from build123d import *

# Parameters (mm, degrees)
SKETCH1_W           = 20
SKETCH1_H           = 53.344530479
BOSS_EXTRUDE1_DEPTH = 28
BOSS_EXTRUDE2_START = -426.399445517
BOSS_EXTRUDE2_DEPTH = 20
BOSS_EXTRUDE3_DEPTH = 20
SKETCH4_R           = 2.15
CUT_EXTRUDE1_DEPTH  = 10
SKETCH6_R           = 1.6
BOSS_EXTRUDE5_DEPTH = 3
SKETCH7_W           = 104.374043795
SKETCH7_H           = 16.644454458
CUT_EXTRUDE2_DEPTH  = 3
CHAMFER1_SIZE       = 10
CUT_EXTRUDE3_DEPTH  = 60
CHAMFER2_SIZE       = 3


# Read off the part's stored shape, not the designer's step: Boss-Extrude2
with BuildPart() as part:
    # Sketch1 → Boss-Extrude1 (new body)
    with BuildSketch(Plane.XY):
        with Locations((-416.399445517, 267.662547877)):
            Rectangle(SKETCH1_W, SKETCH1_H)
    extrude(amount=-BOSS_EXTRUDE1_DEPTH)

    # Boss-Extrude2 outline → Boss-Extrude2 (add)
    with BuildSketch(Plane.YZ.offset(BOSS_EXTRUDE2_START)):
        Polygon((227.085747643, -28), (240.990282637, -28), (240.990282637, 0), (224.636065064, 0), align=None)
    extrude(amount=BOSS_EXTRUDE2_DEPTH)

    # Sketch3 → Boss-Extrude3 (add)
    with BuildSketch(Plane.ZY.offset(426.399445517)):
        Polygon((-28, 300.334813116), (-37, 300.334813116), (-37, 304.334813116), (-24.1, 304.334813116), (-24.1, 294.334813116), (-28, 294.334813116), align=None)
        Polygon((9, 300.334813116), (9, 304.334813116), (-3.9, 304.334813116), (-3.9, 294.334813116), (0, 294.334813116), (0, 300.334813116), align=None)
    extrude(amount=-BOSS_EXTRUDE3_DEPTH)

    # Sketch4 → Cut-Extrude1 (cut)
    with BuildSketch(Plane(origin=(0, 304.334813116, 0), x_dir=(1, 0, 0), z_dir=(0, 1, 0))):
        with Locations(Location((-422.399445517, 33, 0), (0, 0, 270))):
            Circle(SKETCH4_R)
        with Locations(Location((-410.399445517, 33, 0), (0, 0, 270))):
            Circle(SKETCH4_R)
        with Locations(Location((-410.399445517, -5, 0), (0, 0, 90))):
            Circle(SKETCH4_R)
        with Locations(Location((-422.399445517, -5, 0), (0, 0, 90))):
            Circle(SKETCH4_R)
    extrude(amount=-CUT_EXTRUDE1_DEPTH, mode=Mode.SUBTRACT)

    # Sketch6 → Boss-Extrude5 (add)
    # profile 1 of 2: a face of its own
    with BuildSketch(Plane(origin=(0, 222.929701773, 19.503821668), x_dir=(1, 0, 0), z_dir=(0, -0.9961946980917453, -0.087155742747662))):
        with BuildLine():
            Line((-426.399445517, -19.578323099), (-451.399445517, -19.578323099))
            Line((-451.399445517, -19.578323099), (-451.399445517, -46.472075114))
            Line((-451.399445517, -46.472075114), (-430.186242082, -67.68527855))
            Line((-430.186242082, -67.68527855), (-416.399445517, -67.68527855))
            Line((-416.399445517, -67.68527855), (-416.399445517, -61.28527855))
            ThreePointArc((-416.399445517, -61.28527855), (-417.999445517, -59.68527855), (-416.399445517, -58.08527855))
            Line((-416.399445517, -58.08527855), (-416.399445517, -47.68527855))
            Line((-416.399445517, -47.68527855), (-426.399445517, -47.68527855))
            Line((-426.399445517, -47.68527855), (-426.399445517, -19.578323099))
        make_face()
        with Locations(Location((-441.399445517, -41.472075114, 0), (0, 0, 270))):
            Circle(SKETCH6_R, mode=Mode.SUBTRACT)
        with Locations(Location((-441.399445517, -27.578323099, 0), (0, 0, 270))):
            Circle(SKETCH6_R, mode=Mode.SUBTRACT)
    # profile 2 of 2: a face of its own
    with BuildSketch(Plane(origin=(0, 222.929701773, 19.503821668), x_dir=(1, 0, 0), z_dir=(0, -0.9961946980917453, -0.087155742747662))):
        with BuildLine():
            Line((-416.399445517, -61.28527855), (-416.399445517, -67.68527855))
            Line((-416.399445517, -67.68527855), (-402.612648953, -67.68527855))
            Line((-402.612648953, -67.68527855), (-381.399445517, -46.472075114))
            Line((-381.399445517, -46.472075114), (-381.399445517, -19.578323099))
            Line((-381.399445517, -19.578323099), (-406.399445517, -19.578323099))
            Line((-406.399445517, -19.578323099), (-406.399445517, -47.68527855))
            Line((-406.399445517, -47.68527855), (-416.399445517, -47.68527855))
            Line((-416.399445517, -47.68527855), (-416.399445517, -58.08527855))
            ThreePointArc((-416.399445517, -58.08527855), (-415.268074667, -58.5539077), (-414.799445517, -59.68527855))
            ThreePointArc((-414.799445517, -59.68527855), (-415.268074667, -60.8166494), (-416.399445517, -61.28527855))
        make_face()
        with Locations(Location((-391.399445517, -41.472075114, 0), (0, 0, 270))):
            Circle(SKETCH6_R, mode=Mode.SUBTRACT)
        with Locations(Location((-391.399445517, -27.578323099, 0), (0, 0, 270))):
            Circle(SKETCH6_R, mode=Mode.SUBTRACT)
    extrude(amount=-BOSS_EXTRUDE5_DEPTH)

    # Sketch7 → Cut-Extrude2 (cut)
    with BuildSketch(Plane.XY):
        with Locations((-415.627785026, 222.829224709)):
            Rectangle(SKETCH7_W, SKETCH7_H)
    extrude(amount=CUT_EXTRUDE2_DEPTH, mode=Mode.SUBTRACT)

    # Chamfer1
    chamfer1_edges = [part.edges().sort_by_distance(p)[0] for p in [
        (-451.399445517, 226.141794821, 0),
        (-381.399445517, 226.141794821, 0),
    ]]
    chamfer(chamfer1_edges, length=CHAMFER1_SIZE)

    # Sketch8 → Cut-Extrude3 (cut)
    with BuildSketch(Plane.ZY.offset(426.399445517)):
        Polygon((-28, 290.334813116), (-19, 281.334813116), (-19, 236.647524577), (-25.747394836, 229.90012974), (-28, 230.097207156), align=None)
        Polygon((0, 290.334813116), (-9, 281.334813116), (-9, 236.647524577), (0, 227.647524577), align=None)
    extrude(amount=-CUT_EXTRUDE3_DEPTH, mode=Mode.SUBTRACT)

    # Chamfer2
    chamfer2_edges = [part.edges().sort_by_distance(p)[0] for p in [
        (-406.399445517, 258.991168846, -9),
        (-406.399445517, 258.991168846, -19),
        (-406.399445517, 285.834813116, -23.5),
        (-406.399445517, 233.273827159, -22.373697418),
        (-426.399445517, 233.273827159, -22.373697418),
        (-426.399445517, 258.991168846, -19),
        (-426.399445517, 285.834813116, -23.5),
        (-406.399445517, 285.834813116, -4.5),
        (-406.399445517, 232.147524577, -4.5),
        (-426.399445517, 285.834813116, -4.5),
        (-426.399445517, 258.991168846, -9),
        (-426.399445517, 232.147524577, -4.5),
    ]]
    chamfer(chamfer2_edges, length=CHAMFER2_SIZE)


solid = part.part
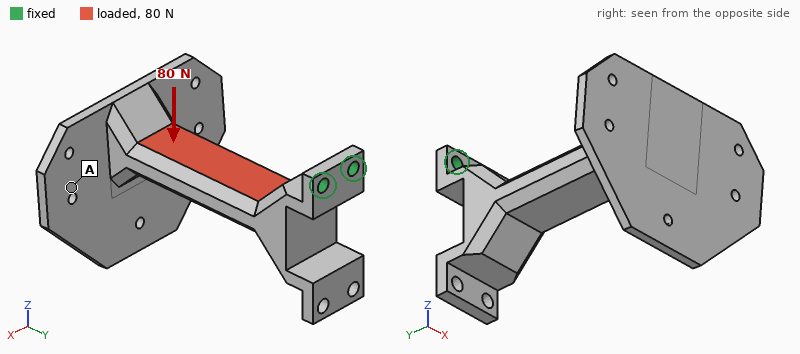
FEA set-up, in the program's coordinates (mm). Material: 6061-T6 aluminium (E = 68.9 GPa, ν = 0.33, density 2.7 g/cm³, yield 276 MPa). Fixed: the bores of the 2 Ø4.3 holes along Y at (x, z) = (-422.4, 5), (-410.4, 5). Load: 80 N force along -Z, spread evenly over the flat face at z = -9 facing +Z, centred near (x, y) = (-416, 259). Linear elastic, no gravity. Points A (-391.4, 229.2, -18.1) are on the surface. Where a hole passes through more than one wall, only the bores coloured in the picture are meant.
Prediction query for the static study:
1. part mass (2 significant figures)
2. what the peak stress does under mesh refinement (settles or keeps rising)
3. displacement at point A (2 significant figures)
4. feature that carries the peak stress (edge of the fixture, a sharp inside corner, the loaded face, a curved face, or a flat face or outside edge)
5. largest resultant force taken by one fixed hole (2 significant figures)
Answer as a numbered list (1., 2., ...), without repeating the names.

1. 73 g
2. keeps rising
3. 0.48 mm
4. edge of the fixture
5. 53 N
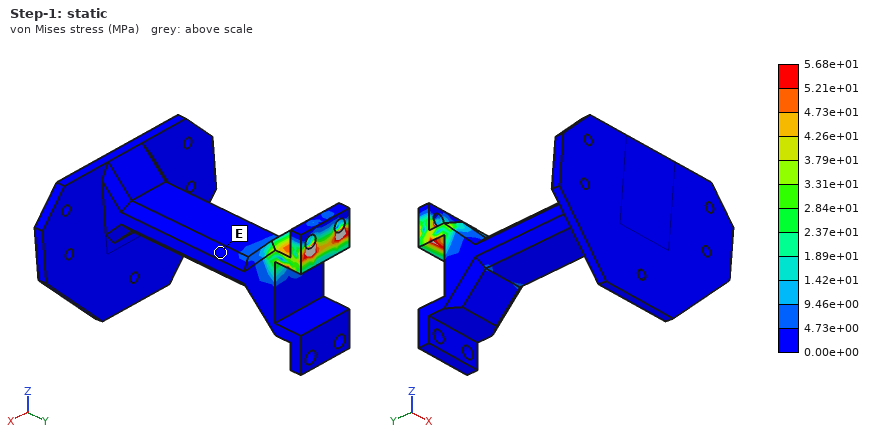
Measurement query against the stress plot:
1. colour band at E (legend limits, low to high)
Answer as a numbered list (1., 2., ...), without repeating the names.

1. 0.00e+00 to 4.73e+00 MPa
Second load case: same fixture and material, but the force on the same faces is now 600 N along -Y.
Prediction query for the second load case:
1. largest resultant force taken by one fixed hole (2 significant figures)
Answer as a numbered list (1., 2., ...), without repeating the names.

1. 300 N
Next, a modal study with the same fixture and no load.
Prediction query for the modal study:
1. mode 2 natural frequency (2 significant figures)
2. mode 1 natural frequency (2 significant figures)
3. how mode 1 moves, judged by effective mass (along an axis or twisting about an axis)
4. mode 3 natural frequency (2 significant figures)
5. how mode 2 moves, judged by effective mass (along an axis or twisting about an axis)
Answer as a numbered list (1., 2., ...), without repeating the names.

1. 700 Hz
2. 240 Hz
3. along Z
4. 1400 Hz
5. along X
